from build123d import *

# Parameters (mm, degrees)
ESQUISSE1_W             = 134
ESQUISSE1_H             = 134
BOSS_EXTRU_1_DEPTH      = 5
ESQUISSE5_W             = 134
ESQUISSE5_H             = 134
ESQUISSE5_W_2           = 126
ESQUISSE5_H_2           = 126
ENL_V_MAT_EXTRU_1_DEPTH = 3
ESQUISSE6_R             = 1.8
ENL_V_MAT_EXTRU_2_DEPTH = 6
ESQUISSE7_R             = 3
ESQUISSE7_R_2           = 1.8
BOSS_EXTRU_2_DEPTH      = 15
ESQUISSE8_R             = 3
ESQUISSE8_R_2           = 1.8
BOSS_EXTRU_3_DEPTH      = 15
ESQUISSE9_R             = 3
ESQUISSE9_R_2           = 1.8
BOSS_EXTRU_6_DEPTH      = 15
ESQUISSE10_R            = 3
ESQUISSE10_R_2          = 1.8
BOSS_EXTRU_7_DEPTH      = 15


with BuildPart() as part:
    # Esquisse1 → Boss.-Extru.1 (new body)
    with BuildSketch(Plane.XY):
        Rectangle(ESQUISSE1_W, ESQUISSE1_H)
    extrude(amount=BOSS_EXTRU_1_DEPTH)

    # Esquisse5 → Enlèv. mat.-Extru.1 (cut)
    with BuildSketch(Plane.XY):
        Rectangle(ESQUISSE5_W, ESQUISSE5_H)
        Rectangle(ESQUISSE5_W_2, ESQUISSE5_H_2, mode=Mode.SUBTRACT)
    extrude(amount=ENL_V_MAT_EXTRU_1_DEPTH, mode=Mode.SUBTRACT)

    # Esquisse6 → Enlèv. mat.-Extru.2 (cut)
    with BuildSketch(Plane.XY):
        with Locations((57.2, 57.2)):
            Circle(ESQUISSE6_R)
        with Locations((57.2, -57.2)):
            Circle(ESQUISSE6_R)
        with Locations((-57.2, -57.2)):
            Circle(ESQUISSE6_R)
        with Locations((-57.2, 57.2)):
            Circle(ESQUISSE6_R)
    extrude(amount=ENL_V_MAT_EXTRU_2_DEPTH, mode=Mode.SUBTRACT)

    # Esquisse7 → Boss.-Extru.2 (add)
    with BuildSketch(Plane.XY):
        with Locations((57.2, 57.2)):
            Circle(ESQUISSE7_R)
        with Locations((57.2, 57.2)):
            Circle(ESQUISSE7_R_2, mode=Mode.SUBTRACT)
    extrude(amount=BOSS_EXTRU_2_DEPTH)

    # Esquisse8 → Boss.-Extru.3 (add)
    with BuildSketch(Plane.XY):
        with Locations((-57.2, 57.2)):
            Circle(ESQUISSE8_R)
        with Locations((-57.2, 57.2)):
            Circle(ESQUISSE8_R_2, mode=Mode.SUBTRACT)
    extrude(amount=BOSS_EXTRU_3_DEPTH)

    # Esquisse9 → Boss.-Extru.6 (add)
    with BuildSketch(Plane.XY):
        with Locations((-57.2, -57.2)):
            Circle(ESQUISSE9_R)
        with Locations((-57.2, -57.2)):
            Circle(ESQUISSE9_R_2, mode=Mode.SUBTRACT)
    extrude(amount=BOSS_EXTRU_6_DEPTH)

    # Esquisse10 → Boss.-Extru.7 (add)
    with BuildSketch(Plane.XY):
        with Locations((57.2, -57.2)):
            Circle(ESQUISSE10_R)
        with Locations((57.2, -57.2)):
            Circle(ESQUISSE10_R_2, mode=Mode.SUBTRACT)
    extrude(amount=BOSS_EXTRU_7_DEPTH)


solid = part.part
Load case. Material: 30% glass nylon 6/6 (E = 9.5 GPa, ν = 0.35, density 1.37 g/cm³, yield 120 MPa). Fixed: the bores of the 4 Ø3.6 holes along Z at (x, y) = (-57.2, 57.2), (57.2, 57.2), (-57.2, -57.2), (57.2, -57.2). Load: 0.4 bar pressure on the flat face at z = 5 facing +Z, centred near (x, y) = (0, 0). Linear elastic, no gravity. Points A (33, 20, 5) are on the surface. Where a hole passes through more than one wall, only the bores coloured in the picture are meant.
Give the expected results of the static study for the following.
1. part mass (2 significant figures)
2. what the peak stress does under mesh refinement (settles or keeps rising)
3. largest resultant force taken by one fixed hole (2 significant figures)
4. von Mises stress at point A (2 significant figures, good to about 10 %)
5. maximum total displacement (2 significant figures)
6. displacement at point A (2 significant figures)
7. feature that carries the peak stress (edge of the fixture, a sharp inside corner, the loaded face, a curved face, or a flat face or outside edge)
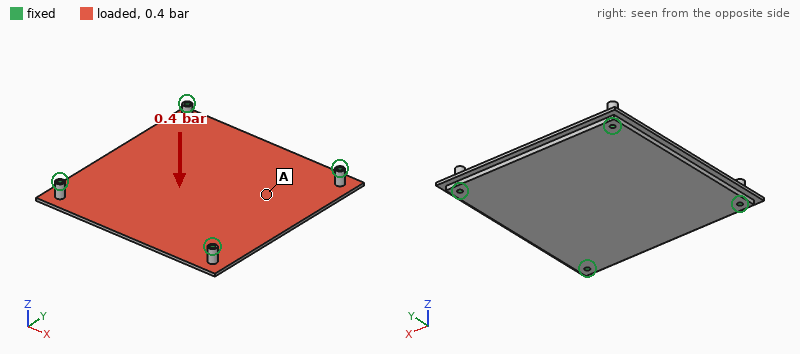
120 g
keeps rising
180 N
5.6 MPa
0.57 mm
0.41 mm
edge of the fixture
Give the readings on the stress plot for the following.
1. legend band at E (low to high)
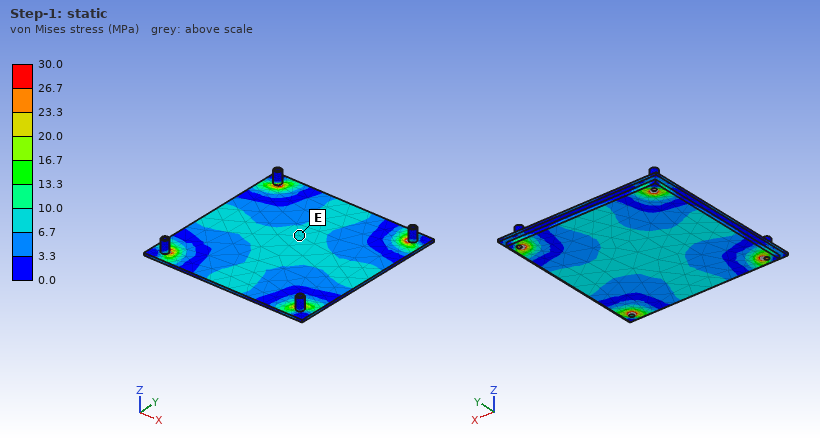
6.7 to 10.0 MPa
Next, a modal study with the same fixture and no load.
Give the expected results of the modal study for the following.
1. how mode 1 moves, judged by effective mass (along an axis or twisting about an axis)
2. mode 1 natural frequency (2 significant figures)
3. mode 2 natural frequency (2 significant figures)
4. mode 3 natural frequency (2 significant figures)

along Z
620 Hz
1100 Hz
1100 Hz
